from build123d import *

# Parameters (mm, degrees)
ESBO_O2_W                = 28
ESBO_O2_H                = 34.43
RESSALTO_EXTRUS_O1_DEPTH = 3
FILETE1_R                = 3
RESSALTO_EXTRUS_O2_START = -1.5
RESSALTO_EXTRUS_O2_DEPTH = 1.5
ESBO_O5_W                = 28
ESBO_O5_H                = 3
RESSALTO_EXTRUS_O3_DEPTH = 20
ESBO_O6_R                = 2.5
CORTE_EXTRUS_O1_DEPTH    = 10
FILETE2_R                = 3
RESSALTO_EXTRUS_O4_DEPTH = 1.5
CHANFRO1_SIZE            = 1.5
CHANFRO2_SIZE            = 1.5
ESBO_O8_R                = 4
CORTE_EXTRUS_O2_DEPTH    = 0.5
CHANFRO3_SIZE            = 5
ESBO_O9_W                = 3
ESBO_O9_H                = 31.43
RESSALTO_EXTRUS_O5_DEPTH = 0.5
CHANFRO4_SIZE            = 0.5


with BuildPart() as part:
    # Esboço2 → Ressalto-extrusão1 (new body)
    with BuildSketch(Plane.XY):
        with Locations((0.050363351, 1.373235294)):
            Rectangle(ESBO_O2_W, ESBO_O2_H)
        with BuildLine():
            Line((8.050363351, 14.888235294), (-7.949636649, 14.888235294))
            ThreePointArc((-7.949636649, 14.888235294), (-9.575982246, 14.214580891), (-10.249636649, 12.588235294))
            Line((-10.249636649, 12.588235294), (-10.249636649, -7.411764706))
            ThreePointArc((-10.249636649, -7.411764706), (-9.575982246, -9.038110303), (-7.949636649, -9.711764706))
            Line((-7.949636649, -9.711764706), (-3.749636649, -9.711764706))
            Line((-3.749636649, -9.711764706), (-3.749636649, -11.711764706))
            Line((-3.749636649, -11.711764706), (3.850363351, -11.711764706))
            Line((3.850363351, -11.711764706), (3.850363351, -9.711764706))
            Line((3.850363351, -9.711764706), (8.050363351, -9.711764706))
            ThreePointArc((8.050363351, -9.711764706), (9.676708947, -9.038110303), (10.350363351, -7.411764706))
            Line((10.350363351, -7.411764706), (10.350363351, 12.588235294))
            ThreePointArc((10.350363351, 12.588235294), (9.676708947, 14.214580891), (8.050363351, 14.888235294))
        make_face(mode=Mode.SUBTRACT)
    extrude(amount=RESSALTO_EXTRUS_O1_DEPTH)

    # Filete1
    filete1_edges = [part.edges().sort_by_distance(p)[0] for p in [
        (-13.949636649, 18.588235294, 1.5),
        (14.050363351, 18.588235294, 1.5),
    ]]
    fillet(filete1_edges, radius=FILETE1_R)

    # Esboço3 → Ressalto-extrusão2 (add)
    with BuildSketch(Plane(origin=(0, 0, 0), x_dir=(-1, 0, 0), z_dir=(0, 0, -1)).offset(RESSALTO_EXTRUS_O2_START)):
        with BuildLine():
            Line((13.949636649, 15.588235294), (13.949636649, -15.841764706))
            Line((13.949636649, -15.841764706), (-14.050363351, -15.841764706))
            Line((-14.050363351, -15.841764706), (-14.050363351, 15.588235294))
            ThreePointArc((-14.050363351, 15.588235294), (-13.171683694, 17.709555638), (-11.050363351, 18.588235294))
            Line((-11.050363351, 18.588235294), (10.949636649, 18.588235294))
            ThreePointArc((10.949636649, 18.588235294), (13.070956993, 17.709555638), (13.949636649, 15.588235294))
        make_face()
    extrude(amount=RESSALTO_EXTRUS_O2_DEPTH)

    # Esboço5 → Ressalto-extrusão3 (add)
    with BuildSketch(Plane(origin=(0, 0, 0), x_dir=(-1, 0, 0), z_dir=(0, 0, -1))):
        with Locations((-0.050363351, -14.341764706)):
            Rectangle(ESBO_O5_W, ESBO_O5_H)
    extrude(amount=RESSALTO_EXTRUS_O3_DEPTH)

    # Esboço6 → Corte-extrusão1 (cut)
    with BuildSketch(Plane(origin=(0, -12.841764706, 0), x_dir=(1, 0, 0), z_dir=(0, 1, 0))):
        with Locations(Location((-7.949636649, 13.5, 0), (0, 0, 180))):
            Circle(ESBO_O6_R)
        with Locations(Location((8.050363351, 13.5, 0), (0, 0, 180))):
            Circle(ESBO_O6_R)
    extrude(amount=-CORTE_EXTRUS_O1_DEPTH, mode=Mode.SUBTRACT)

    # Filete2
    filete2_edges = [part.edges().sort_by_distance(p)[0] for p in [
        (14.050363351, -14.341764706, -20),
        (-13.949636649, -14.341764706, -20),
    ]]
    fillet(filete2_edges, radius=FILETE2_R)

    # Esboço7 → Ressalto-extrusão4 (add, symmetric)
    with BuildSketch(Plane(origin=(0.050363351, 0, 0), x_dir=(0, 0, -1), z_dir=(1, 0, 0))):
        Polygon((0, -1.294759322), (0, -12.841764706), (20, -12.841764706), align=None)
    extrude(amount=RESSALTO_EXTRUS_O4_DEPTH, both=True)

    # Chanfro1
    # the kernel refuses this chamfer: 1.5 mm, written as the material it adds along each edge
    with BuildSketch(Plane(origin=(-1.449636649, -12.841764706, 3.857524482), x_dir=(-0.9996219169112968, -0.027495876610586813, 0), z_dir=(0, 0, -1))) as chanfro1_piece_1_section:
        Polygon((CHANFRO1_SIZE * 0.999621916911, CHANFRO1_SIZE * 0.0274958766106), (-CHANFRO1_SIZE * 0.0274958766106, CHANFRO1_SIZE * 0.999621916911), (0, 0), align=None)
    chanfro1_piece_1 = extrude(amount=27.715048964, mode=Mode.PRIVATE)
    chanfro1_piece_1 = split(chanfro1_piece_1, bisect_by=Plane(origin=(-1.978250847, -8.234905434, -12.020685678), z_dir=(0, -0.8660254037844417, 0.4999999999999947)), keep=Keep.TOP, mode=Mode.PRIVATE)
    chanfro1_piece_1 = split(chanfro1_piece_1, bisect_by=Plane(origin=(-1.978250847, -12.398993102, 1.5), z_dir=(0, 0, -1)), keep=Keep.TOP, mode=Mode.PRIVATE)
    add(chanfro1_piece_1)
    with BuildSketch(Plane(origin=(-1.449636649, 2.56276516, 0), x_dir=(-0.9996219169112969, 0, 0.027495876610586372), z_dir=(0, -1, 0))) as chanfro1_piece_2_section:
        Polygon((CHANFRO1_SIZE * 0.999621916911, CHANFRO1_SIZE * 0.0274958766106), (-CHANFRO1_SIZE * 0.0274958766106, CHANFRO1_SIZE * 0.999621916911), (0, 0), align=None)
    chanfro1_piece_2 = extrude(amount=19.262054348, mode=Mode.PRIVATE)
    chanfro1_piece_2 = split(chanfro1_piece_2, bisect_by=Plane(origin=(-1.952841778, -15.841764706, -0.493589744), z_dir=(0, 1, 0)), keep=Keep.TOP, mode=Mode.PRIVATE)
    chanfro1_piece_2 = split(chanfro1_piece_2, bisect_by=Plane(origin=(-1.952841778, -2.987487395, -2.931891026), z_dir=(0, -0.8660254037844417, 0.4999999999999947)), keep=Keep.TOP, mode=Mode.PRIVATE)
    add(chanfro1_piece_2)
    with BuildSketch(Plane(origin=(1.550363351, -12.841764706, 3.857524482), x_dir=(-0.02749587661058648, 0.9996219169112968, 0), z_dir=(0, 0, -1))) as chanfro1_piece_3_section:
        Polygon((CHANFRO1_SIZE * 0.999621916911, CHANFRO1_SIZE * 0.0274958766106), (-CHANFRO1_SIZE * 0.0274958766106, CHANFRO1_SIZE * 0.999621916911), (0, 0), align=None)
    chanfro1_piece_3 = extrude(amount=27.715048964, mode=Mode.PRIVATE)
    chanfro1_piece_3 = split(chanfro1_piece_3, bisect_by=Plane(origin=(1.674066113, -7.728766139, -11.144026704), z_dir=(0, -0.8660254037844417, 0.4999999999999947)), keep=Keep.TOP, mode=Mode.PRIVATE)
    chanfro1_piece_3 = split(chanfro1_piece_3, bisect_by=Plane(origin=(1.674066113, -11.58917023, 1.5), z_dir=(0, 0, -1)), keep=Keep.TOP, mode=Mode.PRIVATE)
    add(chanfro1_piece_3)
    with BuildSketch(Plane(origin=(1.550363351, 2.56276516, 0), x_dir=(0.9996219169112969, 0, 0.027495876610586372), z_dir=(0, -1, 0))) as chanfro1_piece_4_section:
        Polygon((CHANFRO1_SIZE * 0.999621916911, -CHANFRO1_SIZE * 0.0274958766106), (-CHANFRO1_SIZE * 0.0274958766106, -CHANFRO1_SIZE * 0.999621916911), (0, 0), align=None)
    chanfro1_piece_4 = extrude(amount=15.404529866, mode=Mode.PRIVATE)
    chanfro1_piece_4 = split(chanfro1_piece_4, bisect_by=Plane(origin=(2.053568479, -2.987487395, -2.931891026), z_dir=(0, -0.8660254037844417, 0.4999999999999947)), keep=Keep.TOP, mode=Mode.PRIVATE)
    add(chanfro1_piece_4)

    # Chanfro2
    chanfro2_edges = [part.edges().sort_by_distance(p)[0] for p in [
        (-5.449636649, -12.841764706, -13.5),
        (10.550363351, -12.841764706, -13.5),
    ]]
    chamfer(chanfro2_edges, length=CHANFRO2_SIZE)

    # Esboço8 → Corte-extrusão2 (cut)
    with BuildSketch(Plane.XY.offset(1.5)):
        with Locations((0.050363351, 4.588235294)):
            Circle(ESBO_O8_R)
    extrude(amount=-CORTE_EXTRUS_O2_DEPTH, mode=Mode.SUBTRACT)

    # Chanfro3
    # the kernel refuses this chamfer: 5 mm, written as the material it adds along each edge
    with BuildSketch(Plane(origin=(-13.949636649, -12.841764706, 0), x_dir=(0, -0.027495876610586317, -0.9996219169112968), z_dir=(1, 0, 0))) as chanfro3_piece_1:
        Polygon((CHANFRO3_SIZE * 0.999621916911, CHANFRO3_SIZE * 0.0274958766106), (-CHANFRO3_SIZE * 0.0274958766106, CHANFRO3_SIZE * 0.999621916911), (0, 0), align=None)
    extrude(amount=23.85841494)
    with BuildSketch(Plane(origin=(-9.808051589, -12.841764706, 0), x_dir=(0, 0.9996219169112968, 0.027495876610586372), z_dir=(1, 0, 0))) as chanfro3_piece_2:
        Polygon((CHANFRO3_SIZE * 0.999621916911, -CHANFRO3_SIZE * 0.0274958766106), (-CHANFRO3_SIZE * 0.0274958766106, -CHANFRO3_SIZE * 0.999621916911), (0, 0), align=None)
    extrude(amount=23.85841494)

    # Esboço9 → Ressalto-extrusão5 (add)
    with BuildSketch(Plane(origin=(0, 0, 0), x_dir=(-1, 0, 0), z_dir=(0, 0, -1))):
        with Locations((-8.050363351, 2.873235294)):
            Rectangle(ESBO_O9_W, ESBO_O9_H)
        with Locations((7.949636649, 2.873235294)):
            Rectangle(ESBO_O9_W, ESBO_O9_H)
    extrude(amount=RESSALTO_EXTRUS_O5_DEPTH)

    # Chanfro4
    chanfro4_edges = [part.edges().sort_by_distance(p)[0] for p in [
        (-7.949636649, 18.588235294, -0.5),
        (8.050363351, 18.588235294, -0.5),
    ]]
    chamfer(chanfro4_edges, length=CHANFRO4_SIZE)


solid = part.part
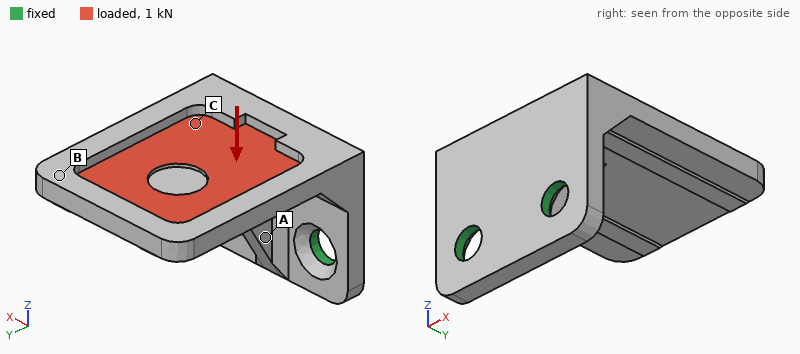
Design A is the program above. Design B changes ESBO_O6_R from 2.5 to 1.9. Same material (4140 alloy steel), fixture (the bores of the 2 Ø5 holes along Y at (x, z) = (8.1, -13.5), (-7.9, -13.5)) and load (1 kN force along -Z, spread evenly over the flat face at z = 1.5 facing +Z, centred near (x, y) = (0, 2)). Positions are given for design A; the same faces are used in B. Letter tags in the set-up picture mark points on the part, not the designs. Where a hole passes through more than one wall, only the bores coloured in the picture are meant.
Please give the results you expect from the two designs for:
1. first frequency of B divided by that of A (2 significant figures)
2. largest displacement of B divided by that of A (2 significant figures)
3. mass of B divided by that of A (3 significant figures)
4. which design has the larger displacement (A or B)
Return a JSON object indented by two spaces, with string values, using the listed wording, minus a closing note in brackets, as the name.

{
  "first frequency of B divided by that of A": "0.94",
  "largest displacement of B divided by that of A": "1.1",
  "mass of B divided by that of A": "1.01",
  "which design has the larger displacement": "B"
}
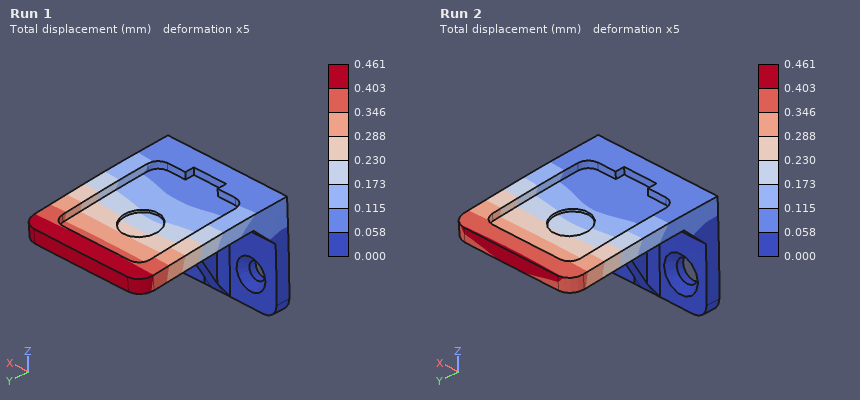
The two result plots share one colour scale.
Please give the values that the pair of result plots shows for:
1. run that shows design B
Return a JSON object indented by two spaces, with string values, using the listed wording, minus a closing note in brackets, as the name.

{
  "run that shows design B": "Run 1"
}
